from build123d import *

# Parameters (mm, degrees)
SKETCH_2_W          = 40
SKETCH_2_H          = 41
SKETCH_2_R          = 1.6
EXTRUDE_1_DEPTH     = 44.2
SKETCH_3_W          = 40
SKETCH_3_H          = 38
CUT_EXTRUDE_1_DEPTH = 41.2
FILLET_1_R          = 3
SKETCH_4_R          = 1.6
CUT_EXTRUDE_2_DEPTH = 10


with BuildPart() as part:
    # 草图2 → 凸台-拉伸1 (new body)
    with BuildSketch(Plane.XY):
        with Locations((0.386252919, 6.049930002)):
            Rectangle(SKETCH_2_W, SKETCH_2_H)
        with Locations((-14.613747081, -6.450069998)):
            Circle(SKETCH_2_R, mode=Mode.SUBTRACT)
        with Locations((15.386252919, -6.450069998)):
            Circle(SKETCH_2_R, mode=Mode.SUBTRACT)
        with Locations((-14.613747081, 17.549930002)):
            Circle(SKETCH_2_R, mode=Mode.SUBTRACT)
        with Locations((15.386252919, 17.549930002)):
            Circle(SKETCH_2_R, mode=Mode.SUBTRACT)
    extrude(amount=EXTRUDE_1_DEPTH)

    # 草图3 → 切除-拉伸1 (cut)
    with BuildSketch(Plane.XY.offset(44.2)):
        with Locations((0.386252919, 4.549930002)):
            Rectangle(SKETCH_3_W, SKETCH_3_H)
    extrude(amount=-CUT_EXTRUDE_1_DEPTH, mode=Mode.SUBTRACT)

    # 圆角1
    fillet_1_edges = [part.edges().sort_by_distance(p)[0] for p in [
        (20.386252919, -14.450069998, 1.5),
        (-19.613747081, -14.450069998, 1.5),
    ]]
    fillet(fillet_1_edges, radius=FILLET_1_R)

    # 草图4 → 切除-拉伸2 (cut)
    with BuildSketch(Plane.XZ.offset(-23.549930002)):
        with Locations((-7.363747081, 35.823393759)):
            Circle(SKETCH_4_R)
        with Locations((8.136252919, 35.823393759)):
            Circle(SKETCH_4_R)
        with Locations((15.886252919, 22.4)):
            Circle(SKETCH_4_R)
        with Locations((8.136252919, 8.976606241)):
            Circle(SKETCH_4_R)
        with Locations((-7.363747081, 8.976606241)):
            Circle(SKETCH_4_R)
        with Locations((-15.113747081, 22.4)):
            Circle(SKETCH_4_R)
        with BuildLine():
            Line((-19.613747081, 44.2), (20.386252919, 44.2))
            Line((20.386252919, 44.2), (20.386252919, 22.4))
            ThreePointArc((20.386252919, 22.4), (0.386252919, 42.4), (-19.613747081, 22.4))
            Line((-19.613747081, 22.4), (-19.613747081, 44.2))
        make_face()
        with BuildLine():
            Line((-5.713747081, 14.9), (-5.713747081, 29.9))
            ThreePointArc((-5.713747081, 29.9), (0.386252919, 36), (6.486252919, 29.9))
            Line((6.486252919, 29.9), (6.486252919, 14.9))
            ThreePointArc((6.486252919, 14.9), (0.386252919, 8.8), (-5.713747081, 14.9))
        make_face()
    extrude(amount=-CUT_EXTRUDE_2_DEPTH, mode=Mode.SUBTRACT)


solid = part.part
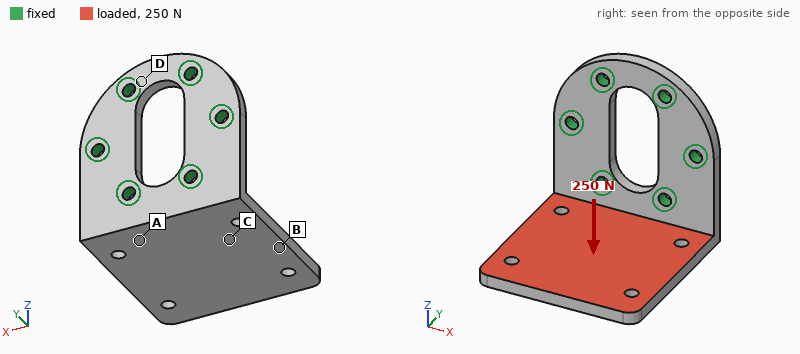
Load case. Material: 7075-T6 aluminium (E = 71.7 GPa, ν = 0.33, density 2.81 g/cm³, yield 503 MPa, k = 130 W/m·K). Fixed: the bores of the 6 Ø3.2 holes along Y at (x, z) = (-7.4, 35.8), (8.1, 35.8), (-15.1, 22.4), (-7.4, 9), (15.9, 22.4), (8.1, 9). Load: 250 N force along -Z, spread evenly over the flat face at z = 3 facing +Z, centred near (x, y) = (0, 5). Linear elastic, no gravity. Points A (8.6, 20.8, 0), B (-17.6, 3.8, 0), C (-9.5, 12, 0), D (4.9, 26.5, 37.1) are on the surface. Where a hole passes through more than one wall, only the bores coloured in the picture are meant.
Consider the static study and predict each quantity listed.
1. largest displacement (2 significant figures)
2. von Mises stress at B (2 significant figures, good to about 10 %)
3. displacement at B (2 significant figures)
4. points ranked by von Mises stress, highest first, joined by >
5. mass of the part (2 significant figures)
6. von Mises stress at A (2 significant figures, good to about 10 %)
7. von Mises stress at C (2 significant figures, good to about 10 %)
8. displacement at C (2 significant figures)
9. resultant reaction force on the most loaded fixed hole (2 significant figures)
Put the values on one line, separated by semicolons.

0.52 mm; 18 MPa; 0.24 mm; A > C > B > D; 22 g; 63 MPa; 35 MPa; 0.13 mm; 130 N
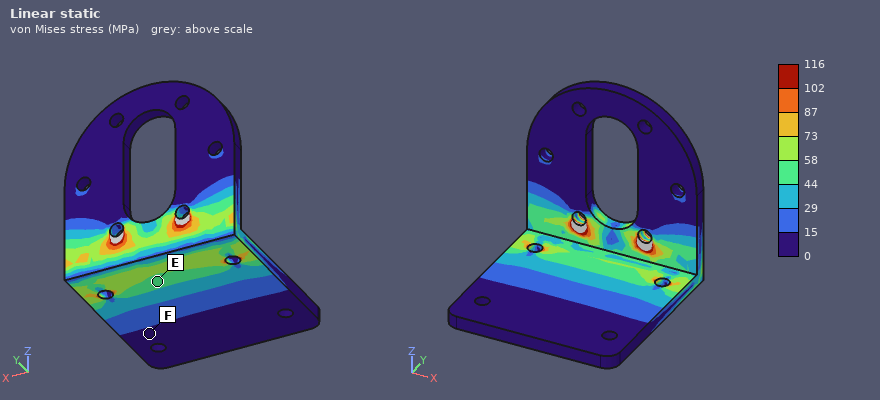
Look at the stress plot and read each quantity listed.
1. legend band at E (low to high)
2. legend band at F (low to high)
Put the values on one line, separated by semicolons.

44 to 58 MPa; 0 to 15 MPa
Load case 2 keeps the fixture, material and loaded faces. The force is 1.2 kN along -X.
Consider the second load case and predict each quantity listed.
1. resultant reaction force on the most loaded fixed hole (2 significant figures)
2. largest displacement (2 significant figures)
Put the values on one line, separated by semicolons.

1.4 kN; 0.29 mm
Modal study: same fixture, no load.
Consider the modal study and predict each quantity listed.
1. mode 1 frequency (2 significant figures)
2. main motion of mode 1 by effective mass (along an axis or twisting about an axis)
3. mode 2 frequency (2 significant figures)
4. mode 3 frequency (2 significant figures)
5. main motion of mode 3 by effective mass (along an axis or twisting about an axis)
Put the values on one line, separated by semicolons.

1200 Hz; along Z; 3100 Hz; 4300 Hz; along X
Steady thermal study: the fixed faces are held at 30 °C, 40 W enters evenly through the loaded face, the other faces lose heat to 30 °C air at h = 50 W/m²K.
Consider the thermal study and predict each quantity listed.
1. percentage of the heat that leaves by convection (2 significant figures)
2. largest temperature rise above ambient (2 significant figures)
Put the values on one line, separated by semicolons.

14 %; 65 K
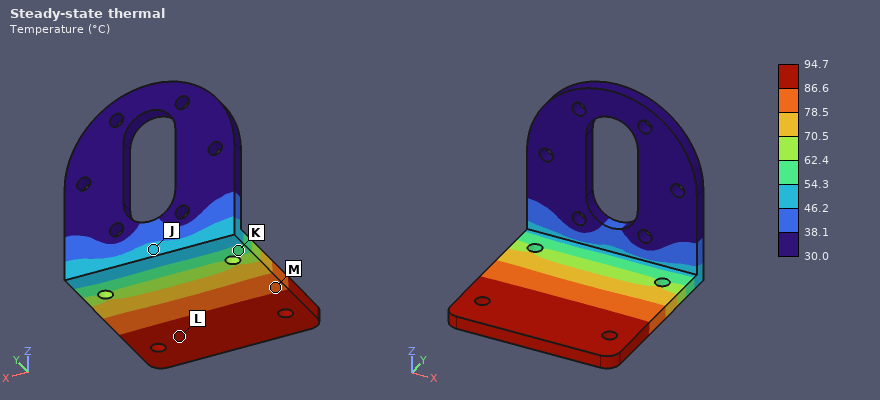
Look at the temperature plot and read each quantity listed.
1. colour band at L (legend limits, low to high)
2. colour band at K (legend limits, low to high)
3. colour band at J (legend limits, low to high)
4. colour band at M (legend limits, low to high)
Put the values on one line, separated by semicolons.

86.6 to 94.7 °C; 54.3 to 62.4 °C; 46.2 to 54.3 °C; 78.5 to 86.6 °C
